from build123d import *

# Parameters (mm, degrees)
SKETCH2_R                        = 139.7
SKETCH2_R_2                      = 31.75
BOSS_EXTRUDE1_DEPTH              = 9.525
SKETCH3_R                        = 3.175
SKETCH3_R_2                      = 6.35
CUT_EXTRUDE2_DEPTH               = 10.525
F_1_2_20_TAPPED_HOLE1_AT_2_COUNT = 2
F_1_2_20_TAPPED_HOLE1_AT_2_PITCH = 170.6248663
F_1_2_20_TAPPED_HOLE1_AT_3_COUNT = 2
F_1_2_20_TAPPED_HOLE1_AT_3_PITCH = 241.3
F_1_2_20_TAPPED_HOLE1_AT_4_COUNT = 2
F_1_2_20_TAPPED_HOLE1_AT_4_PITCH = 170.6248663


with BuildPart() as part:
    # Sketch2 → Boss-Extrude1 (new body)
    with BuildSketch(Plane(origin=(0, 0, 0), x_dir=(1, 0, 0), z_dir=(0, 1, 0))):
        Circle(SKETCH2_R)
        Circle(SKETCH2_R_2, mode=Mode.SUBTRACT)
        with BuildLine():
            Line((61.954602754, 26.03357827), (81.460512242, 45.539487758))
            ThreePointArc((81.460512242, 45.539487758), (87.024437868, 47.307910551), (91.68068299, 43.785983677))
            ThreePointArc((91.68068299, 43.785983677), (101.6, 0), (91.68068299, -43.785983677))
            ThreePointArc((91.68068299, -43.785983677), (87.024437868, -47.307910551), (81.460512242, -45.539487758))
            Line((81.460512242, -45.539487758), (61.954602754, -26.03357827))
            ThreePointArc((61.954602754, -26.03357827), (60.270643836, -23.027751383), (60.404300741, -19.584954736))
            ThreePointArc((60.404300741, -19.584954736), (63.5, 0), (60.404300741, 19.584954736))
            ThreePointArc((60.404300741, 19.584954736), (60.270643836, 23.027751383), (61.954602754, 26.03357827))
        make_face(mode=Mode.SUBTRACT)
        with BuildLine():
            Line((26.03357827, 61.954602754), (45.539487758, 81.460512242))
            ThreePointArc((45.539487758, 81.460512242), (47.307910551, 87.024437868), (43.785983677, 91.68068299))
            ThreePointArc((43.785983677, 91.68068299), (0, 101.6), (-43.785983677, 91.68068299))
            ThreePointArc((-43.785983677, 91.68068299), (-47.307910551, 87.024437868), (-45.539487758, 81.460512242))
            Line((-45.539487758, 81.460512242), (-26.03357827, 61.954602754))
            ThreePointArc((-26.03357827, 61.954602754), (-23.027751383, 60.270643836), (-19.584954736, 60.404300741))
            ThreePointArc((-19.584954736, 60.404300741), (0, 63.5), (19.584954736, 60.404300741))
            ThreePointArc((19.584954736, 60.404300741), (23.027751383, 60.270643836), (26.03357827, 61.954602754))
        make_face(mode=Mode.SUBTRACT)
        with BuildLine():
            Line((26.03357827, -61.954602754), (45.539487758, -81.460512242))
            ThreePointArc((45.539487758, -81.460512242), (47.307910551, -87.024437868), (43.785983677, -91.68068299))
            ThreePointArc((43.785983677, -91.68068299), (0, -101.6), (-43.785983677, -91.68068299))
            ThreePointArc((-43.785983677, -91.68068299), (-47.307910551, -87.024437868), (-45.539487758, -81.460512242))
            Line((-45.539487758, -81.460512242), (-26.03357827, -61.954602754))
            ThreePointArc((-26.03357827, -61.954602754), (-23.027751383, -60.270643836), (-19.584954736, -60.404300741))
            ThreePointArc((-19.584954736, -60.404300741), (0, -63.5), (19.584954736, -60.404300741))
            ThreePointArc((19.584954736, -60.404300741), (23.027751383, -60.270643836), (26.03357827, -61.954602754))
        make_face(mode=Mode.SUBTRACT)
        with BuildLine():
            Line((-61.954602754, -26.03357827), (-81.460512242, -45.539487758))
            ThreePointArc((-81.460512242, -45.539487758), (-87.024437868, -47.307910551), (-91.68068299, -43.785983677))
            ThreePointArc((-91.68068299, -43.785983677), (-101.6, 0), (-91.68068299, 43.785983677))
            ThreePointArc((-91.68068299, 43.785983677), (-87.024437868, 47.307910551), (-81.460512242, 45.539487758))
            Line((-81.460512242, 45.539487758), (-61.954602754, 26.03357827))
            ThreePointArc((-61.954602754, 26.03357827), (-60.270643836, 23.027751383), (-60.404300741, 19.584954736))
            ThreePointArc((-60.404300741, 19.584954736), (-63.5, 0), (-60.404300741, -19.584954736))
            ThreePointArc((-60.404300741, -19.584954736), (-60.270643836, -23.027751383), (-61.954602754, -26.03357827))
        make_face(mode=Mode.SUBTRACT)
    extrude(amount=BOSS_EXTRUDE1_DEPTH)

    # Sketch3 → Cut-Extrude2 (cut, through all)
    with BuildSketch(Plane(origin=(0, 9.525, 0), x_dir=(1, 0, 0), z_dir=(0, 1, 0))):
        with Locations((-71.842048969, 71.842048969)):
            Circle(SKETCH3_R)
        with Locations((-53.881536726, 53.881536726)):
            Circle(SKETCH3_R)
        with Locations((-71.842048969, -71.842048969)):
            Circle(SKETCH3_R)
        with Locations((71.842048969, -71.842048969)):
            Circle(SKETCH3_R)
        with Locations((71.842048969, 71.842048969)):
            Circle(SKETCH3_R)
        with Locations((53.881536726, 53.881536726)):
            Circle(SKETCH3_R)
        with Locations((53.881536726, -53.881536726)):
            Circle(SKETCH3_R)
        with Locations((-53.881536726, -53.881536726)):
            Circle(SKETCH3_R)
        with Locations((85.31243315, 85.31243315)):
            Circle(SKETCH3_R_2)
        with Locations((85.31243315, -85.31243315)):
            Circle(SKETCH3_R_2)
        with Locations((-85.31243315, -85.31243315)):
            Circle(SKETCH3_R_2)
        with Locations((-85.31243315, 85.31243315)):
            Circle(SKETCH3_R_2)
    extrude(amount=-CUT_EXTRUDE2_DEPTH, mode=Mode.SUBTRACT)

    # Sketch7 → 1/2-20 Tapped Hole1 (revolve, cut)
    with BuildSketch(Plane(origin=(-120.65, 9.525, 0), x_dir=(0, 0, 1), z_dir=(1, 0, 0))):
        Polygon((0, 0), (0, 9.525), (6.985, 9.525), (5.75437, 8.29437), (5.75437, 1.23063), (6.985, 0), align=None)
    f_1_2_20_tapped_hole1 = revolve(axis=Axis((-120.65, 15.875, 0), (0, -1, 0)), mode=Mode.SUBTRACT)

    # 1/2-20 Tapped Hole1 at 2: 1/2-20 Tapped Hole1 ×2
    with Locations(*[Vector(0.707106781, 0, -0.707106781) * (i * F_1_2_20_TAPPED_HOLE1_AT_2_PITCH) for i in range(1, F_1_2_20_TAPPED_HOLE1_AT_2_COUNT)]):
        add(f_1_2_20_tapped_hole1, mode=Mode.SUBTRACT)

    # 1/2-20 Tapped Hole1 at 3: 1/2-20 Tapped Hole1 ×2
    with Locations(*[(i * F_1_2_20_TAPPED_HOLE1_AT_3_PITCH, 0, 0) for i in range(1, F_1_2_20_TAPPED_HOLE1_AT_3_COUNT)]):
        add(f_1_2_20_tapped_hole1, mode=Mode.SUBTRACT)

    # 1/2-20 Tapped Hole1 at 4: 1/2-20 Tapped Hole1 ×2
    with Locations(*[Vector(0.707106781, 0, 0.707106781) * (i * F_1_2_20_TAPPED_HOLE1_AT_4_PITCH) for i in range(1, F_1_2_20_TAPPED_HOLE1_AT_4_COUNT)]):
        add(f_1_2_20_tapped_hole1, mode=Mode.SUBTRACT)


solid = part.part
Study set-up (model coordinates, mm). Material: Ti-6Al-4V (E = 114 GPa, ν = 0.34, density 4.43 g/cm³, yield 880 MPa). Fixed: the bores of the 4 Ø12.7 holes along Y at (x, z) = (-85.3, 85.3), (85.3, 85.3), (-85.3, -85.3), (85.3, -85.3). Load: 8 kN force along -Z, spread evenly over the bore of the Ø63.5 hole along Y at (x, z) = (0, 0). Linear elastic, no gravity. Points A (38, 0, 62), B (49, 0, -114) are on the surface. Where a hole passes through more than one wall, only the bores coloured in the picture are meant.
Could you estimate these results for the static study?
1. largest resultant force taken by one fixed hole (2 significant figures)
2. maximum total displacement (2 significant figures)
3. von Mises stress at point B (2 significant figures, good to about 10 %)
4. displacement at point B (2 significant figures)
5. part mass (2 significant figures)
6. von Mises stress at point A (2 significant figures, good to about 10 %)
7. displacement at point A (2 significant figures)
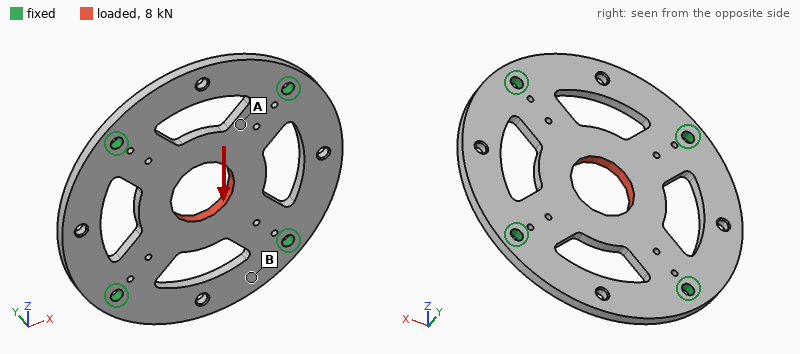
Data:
2.2 kN
8.1 µm
1.9 MPa
2.1 µm
1.9 kg
5.4 MPa
4.5 µm
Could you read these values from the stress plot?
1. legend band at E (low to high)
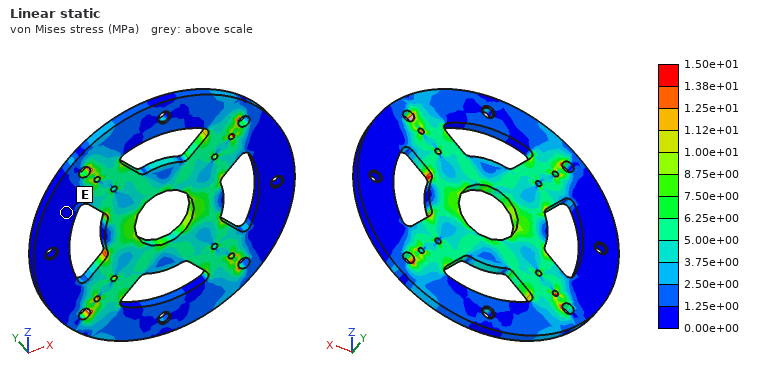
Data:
0.00e+00 to 1.25e+00 MPa
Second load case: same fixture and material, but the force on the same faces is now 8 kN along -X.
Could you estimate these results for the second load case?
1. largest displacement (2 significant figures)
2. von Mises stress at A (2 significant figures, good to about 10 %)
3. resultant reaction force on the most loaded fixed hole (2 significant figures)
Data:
8.1 µm
5.9 MPa
2.2 kN
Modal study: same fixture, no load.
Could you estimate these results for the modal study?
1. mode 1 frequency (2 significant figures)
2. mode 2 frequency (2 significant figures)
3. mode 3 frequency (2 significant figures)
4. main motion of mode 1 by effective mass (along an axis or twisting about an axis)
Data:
1200 Hz
1400 Hz
1400 Hz
along Y
